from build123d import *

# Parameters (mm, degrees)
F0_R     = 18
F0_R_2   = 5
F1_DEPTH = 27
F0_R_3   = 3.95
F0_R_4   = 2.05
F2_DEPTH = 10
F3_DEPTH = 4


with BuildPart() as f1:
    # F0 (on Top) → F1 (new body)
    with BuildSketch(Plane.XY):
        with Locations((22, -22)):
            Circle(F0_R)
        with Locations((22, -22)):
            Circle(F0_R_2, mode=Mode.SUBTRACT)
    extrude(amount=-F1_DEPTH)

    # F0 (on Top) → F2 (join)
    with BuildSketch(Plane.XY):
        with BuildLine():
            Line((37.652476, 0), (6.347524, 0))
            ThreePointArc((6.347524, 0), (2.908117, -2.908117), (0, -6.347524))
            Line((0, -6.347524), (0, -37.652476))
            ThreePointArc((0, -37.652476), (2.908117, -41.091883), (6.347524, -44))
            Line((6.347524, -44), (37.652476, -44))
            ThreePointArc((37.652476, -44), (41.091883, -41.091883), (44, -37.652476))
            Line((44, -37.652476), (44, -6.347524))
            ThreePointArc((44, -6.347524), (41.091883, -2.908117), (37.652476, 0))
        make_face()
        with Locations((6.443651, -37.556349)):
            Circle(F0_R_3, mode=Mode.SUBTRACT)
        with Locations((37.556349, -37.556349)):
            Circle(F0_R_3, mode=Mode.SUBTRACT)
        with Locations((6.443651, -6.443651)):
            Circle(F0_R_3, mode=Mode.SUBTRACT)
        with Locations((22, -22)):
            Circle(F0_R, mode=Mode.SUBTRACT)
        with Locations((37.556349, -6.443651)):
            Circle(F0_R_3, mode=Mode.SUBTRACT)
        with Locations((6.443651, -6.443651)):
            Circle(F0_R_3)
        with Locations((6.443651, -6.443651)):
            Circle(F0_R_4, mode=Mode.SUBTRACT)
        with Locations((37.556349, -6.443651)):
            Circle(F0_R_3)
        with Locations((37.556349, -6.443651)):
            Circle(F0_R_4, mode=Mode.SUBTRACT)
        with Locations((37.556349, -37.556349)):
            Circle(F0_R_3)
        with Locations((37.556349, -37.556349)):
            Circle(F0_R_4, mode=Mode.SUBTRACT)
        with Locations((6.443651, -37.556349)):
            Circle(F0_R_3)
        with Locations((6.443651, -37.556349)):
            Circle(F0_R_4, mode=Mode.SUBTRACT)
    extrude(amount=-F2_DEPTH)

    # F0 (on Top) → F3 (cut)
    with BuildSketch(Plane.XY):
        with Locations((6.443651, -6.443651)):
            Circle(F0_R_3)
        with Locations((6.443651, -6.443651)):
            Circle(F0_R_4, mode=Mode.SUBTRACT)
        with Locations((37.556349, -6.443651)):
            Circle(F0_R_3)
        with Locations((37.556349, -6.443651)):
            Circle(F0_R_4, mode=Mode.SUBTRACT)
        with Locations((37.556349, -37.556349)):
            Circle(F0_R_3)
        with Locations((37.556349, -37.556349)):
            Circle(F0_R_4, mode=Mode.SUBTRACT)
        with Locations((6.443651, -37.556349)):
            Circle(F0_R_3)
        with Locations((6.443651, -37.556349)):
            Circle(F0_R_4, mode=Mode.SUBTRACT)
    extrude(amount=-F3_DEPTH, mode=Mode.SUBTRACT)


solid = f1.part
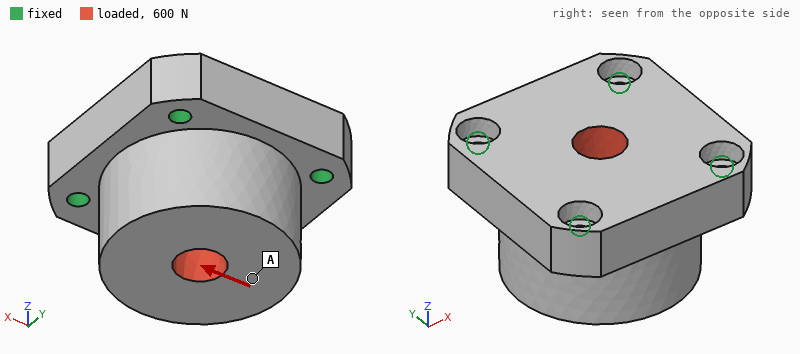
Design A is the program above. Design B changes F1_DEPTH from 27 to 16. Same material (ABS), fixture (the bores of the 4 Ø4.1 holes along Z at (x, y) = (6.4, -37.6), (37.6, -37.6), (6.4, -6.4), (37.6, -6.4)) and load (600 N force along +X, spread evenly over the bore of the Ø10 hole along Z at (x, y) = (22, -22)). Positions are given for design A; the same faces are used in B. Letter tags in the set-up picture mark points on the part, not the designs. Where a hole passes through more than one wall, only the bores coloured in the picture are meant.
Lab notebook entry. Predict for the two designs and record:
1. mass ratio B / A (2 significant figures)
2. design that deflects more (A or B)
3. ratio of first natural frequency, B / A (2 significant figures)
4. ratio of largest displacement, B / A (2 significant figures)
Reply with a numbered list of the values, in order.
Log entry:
1. 0.68
2. A
3. 1.3
4. 0.61
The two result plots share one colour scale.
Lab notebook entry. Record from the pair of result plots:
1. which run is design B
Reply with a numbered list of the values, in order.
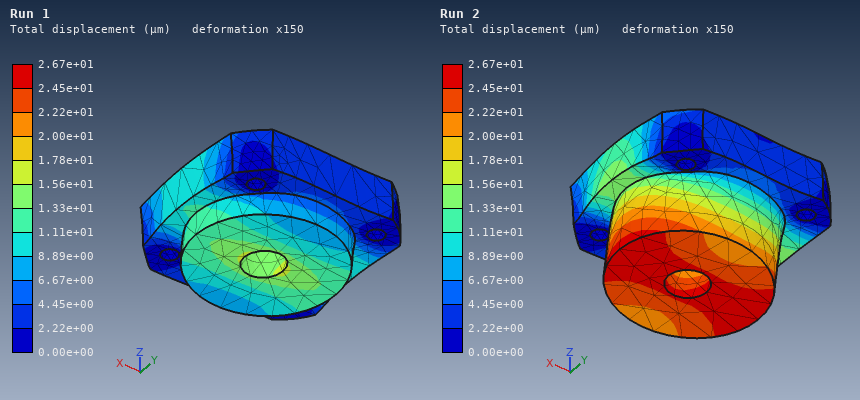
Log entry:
1. Run 1
